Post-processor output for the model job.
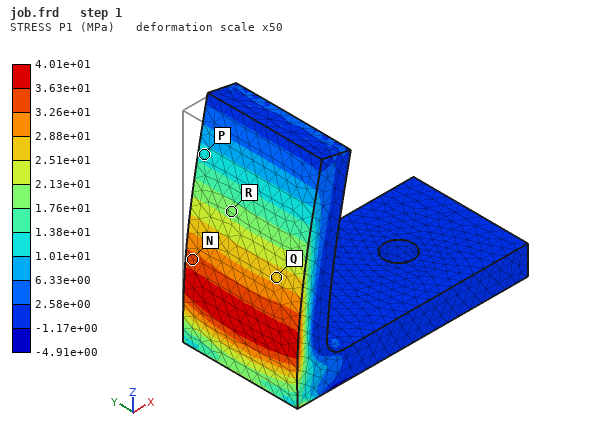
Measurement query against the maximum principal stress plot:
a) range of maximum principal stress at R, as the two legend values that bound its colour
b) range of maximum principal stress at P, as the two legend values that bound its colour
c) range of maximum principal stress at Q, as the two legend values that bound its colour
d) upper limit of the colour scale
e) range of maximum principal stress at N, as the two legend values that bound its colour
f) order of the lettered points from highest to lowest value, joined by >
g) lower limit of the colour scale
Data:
1.76e+01 to 2.13e+01 MPa
1.01e+01 to 1.38e+01 MPa
2.51e+01 to 2.88e+01 MPa
4.01e+01 MPa
3.26e+01 to 3.63e+01 MPa
N > Q > R > P
-4.91e+00 MPa
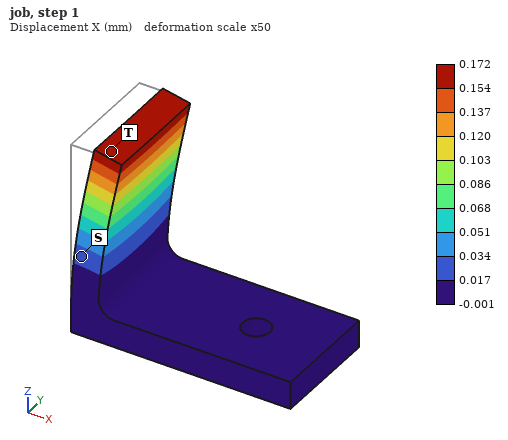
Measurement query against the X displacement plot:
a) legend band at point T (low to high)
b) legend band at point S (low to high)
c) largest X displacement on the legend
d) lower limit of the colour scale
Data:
0.154 to 0.172 mm
0.017 to 0.034 mm
0.172 mm
-0.001 mm
